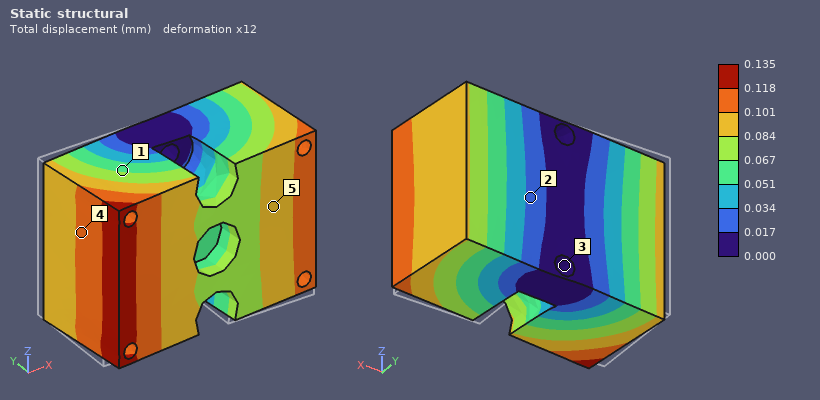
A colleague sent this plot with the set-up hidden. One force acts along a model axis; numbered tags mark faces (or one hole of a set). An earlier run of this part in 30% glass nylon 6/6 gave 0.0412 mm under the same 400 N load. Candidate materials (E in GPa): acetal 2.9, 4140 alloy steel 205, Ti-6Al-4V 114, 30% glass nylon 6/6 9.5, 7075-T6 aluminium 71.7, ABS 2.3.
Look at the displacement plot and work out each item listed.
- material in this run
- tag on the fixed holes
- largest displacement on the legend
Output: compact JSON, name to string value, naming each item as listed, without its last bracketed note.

{"material in this run": "acetal", "tag on the fixed holes": "3", "largest displacement on the legend": "0.135 mm"}
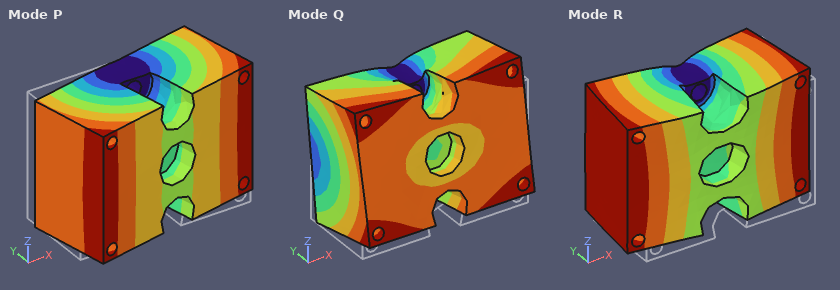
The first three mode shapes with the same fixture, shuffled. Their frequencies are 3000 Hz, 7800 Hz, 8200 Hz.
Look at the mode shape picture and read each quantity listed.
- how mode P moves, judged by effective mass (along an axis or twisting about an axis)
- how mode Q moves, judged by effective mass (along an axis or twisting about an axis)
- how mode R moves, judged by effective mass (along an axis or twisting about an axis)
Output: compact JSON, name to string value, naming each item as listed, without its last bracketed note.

{"how mode P moves, judged by effective mass": "along X", "how mode Q moves, judged by effective mass": "along Z", "how mode R moves, judged by effective mass": "along Y"}
